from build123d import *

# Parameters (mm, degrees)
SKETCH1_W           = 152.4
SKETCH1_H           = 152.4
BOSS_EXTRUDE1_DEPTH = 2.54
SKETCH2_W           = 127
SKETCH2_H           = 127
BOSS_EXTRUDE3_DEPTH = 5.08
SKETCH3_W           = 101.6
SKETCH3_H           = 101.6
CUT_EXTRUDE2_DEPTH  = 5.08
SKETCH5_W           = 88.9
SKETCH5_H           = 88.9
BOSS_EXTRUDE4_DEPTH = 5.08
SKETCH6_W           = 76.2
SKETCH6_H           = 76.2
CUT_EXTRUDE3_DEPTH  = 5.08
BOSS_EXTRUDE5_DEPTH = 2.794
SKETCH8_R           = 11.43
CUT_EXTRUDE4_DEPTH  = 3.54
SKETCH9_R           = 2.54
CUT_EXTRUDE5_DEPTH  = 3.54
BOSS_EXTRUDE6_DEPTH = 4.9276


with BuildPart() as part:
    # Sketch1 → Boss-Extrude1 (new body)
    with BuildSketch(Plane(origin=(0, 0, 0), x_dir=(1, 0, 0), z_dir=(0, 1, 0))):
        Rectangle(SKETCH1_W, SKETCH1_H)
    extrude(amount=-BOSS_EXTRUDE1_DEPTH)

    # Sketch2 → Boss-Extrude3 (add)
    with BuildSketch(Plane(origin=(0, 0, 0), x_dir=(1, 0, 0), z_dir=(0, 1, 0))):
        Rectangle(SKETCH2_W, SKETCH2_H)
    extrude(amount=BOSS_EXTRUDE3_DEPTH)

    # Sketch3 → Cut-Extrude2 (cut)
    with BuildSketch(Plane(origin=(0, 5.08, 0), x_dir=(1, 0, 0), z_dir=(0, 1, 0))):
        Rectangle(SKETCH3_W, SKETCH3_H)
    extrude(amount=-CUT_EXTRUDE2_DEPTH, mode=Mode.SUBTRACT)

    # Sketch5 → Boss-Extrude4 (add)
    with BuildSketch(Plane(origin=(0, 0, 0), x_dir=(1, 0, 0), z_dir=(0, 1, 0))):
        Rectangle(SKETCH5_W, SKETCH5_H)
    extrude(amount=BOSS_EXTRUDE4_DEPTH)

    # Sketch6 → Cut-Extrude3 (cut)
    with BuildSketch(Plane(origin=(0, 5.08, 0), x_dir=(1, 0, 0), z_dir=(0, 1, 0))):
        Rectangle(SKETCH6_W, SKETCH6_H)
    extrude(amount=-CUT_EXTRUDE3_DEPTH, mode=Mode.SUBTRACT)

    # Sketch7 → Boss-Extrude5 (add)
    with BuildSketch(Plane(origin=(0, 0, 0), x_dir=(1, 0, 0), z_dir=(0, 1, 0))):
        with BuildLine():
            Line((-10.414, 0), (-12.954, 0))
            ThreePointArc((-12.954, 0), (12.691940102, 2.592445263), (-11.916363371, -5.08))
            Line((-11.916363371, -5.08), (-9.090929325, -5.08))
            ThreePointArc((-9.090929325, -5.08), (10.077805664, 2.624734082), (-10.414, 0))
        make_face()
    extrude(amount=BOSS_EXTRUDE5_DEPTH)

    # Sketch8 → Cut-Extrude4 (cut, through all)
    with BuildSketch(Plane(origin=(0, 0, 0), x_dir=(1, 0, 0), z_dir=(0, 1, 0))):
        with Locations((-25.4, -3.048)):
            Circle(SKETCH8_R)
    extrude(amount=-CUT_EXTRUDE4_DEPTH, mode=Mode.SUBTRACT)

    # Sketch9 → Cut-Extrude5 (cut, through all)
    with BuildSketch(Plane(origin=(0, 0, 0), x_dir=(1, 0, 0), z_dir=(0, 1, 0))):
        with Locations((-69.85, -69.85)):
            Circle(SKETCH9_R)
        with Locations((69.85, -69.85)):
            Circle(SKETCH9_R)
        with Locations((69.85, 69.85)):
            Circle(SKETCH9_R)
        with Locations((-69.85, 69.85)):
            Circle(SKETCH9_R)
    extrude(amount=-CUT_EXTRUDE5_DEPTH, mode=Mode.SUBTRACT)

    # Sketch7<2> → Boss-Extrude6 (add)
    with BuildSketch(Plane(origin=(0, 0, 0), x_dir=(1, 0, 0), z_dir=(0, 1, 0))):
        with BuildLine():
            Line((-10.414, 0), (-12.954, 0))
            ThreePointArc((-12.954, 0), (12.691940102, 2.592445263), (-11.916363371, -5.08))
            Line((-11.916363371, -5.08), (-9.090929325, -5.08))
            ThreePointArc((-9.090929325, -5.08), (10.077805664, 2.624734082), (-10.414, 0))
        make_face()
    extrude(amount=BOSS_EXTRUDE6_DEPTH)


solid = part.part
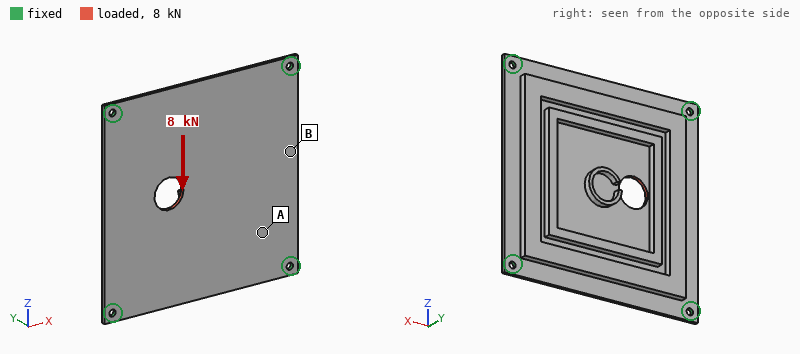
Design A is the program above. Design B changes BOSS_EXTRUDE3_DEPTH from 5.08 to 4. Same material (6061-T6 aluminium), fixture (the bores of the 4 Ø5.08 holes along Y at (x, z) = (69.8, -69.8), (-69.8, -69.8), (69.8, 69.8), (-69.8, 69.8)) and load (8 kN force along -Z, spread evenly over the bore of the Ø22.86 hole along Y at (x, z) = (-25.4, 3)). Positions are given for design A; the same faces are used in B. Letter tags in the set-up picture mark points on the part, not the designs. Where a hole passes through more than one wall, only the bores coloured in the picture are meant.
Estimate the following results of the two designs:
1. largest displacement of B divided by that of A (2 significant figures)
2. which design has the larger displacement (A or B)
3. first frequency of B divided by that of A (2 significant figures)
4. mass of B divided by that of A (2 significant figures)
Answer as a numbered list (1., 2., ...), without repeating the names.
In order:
1. 1.1
2. B
3. 0.90
4. 0.94
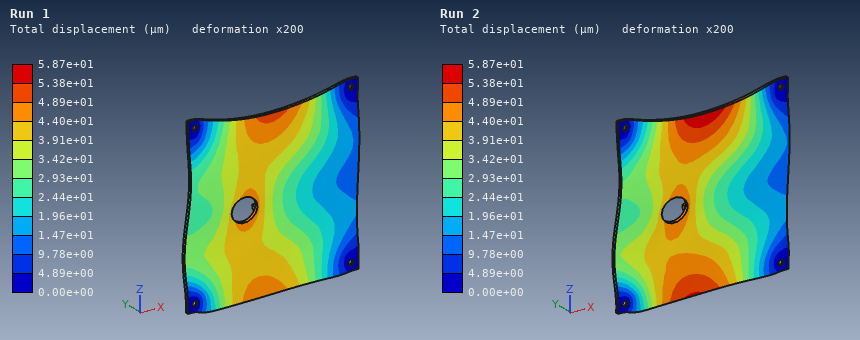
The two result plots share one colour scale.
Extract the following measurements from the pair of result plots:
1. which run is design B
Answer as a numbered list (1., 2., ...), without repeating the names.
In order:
1. Run 2
